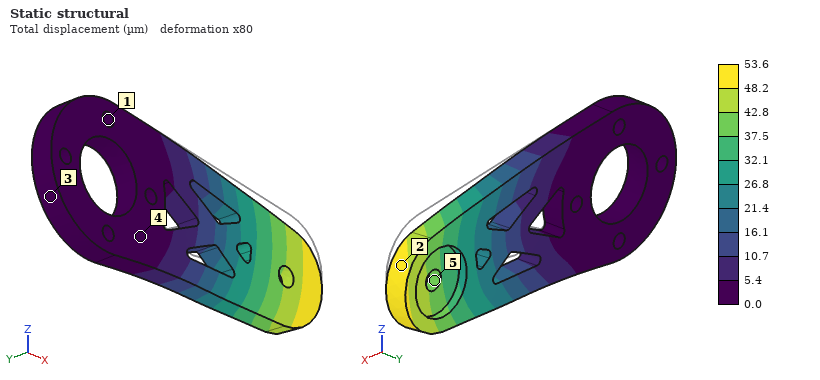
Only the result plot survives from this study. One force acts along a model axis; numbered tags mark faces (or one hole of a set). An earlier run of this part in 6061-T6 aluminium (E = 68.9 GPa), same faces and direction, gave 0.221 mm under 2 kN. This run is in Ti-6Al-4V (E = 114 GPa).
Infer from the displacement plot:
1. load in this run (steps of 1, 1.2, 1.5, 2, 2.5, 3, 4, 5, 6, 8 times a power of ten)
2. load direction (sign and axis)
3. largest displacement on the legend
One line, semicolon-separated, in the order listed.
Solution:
800 N; -Z; 53.6 µm
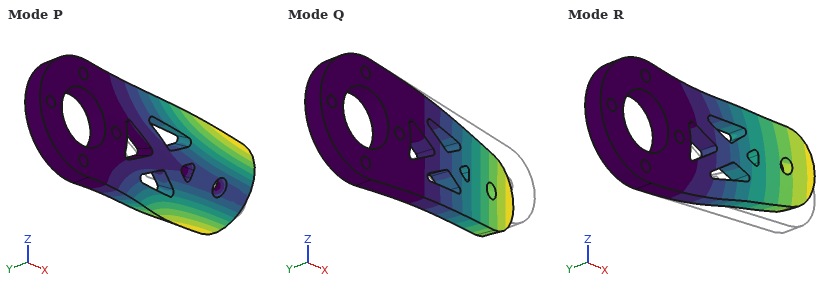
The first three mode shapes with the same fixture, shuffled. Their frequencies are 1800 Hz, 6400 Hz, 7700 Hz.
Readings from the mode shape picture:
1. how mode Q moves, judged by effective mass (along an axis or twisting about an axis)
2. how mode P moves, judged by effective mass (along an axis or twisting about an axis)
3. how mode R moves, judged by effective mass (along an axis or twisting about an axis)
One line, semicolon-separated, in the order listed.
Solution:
along Y; twisting about X; along Z
